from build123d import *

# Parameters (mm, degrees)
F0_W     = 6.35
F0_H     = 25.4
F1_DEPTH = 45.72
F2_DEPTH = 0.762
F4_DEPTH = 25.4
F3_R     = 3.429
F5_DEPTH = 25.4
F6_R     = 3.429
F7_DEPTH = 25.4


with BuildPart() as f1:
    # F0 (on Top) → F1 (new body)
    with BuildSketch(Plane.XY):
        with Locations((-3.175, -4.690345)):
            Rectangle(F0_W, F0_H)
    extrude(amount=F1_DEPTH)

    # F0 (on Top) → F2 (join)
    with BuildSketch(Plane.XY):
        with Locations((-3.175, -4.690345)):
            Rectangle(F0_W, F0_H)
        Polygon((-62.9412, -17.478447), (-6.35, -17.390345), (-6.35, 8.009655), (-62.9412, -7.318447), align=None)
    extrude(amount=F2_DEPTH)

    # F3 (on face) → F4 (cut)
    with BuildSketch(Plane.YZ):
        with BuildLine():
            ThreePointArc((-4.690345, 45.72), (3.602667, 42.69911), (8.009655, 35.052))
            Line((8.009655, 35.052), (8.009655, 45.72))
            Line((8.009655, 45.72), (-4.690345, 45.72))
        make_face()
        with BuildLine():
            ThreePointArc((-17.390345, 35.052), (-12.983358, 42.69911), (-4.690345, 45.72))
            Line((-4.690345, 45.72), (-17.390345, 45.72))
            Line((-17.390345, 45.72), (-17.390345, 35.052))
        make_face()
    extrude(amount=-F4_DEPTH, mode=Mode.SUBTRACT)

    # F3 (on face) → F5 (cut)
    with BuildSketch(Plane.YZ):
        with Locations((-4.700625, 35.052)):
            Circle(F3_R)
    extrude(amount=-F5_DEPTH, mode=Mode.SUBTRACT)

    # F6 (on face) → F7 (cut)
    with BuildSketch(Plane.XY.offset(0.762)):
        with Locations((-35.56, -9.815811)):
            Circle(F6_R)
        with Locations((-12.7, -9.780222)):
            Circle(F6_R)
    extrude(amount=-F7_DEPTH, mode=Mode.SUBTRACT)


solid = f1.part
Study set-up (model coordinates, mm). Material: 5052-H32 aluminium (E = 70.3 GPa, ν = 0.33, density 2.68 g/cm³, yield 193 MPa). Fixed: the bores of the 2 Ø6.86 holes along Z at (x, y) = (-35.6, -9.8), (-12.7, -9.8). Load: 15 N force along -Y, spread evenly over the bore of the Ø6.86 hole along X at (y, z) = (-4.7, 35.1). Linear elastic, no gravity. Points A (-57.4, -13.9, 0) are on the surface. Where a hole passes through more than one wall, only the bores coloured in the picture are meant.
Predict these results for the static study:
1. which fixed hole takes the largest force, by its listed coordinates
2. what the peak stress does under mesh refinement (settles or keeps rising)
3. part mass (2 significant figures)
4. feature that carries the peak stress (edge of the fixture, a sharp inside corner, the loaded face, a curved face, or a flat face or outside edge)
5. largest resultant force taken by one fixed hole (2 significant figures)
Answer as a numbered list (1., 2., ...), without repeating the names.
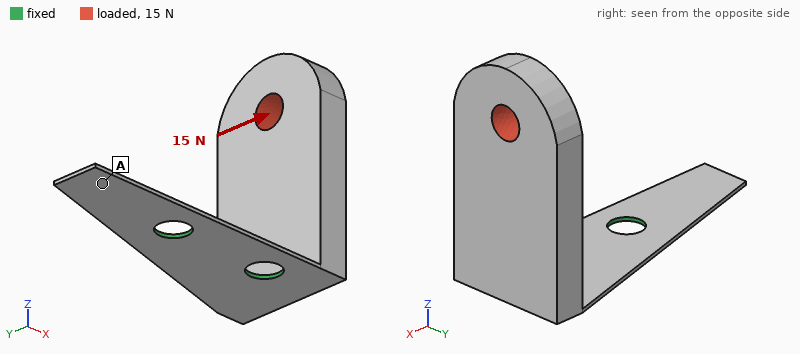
1. (-12.7, -9.8)
2. keeps rising
3. 20 g
4. edge of the fixture
5. 16 N
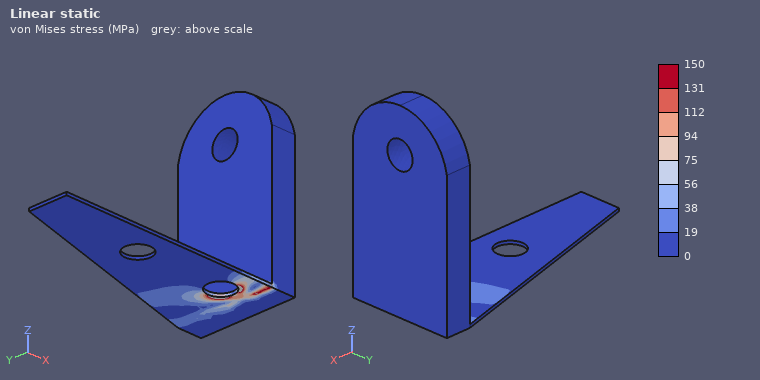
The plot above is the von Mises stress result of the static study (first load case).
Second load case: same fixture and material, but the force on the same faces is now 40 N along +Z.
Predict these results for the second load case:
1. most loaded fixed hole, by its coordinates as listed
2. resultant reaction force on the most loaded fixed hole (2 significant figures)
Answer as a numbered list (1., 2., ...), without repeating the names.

1. (-12.7, -9.8)
2. 41 N
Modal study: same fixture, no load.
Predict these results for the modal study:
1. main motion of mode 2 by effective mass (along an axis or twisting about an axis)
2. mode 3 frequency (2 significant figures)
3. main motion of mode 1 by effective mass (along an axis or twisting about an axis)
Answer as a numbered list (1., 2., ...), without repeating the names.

1. along Y
2. 1200 Hz
3. along X
